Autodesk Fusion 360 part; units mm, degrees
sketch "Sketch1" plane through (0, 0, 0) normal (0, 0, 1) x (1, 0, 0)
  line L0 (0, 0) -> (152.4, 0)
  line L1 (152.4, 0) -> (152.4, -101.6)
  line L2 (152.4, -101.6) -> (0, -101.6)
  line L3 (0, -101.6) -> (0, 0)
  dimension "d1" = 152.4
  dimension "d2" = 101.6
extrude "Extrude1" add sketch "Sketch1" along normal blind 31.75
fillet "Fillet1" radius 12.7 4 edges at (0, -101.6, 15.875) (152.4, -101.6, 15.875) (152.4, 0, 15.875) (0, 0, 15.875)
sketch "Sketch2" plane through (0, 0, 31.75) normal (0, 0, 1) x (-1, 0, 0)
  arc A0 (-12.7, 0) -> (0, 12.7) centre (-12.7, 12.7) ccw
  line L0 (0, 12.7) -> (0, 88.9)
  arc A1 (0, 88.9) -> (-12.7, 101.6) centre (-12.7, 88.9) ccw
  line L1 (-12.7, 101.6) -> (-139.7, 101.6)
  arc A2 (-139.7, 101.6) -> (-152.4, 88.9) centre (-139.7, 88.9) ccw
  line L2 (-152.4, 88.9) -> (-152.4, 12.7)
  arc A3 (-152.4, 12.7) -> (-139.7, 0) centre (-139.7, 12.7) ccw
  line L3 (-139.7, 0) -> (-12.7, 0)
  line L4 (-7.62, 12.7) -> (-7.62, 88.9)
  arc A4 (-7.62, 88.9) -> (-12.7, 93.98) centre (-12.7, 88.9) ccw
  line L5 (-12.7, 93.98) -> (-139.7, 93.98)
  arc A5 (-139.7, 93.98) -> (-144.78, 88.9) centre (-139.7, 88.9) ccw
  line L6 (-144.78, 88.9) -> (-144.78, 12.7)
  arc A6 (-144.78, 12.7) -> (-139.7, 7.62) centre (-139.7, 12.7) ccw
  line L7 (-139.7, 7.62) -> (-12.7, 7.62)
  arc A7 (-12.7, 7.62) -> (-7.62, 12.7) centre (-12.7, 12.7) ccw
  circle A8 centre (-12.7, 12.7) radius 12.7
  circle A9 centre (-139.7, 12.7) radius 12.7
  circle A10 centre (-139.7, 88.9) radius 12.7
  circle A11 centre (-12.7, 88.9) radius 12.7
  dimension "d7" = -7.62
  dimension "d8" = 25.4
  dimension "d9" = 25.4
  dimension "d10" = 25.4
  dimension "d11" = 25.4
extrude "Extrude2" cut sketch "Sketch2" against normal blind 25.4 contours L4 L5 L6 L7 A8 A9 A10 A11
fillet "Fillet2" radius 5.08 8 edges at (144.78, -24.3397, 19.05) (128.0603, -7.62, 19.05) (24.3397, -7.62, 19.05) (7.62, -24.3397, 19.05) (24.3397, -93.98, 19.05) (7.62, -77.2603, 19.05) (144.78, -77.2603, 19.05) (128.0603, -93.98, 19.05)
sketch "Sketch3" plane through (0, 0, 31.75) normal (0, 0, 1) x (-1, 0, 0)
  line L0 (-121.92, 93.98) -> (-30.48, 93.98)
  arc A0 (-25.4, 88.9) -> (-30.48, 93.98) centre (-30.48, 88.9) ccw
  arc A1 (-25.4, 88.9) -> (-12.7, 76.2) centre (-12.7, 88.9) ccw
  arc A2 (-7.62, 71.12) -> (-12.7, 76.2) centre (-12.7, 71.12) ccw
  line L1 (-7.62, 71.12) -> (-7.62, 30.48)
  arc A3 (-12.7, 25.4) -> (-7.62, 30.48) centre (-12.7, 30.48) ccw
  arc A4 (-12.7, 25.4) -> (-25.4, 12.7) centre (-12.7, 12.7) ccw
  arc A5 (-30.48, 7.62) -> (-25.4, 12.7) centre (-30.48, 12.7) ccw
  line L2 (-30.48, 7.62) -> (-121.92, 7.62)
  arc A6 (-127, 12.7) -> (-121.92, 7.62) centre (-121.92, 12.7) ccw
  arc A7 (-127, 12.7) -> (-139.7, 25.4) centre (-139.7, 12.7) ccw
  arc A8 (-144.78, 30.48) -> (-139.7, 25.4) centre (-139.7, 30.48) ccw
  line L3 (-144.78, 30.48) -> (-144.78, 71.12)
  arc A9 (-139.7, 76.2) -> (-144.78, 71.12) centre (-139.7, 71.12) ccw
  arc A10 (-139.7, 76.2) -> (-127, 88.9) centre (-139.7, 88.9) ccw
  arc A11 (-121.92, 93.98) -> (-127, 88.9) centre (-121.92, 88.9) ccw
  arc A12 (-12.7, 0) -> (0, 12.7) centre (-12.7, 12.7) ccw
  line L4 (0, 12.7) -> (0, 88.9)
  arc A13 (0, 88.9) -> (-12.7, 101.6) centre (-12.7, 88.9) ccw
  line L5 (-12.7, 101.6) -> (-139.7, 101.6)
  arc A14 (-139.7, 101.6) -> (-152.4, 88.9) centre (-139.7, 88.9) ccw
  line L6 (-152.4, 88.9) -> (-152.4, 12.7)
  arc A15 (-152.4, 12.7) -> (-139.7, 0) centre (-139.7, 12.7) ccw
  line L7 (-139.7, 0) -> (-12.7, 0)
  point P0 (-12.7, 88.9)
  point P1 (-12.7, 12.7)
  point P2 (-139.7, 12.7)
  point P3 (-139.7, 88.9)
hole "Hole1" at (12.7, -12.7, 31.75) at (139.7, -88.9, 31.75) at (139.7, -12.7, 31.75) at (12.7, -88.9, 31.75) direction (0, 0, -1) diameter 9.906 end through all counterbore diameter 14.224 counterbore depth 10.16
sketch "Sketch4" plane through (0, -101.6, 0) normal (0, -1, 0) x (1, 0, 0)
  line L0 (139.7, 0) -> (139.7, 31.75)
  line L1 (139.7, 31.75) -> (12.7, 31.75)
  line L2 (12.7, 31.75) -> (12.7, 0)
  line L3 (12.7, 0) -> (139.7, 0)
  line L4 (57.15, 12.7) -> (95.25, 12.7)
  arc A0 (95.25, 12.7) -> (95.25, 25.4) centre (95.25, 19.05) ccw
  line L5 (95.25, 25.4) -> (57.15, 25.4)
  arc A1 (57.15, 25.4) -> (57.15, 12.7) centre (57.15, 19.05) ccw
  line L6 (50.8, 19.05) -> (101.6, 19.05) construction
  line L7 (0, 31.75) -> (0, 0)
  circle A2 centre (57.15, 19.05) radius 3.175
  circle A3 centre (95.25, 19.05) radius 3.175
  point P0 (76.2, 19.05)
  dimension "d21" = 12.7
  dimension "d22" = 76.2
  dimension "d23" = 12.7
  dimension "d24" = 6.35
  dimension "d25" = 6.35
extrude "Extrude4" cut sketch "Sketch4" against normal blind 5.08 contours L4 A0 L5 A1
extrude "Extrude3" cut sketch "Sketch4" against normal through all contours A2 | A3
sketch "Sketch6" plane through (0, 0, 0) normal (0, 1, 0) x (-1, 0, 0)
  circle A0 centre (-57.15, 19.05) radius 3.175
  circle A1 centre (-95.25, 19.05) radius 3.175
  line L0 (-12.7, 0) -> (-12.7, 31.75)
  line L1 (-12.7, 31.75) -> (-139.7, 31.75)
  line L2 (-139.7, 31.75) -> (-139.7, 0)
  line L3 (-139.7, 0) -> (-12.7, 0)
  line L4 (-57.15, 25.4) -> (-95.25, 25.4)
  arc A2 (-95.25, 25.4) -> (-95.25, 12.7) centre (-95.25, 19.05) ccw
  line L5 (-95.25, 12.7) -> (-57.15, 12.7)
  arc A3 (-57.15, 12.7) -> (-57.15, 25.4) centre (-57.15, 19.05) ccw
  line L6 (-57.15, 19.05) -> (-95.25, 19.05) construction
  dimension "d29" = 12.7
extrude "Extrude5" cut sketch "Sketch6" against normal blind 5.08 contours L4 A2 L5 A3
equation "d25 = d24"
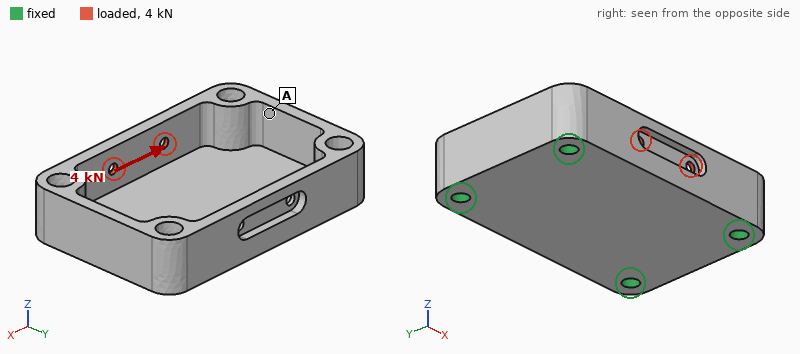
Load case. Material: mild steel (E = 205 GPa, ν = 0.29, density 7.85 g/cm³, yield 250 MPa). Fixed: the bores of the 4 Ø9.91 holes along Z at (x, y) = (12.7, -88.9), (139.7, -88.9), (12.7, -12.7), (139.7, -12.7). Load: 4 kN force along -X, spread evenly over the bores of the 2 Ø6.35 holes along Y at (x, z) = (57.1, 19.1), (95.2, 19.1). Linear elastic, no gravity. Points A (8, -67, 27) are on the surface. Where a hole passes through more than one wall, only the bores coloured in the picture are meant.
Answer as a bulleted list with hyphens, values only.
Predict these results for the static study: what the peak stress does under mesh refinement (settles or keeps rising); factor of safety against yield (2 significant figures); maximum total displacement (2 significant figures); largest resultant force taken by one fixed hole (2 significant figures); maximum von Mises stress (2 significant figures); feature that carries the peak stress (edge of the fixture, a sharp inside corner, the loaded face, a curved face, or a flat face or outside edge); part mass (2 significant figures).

- settles
- 3.4
- 3.2 µm
- 1.9 kN
- 73 MPa
- the loaded face
- 1.5 kg
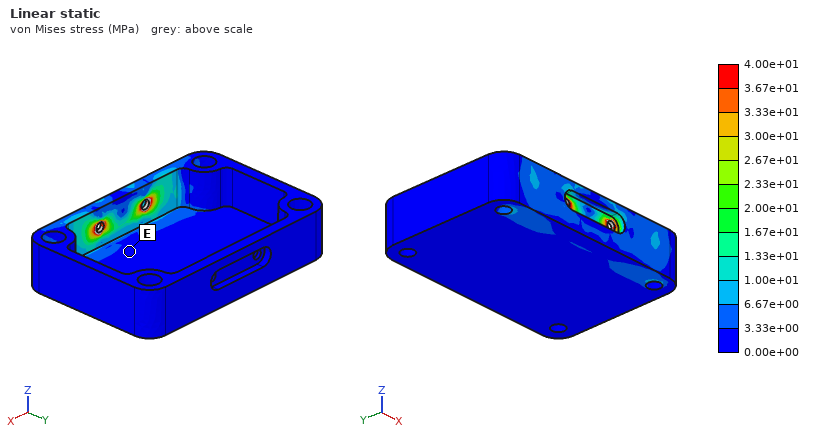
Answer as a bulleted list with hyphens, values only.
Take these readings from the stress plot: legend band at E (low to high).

- 0.00e+00 to 3.33e+00 MPa
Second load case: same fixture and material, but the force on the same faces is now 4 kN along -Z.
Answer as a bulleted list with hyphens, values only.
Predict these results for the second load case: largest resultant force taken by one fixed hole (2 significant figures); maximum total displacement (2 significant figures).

- 2.0 kN
- 13 µm
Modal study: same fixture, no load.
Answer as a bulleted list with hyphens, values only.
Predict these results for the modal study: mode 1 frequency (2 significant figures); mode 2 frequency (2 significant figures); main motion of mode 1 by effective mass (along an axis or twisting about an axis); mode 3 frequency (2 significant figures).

- 3600 Hz
- 6200 Hz
- along Z
- 6600 Hz
